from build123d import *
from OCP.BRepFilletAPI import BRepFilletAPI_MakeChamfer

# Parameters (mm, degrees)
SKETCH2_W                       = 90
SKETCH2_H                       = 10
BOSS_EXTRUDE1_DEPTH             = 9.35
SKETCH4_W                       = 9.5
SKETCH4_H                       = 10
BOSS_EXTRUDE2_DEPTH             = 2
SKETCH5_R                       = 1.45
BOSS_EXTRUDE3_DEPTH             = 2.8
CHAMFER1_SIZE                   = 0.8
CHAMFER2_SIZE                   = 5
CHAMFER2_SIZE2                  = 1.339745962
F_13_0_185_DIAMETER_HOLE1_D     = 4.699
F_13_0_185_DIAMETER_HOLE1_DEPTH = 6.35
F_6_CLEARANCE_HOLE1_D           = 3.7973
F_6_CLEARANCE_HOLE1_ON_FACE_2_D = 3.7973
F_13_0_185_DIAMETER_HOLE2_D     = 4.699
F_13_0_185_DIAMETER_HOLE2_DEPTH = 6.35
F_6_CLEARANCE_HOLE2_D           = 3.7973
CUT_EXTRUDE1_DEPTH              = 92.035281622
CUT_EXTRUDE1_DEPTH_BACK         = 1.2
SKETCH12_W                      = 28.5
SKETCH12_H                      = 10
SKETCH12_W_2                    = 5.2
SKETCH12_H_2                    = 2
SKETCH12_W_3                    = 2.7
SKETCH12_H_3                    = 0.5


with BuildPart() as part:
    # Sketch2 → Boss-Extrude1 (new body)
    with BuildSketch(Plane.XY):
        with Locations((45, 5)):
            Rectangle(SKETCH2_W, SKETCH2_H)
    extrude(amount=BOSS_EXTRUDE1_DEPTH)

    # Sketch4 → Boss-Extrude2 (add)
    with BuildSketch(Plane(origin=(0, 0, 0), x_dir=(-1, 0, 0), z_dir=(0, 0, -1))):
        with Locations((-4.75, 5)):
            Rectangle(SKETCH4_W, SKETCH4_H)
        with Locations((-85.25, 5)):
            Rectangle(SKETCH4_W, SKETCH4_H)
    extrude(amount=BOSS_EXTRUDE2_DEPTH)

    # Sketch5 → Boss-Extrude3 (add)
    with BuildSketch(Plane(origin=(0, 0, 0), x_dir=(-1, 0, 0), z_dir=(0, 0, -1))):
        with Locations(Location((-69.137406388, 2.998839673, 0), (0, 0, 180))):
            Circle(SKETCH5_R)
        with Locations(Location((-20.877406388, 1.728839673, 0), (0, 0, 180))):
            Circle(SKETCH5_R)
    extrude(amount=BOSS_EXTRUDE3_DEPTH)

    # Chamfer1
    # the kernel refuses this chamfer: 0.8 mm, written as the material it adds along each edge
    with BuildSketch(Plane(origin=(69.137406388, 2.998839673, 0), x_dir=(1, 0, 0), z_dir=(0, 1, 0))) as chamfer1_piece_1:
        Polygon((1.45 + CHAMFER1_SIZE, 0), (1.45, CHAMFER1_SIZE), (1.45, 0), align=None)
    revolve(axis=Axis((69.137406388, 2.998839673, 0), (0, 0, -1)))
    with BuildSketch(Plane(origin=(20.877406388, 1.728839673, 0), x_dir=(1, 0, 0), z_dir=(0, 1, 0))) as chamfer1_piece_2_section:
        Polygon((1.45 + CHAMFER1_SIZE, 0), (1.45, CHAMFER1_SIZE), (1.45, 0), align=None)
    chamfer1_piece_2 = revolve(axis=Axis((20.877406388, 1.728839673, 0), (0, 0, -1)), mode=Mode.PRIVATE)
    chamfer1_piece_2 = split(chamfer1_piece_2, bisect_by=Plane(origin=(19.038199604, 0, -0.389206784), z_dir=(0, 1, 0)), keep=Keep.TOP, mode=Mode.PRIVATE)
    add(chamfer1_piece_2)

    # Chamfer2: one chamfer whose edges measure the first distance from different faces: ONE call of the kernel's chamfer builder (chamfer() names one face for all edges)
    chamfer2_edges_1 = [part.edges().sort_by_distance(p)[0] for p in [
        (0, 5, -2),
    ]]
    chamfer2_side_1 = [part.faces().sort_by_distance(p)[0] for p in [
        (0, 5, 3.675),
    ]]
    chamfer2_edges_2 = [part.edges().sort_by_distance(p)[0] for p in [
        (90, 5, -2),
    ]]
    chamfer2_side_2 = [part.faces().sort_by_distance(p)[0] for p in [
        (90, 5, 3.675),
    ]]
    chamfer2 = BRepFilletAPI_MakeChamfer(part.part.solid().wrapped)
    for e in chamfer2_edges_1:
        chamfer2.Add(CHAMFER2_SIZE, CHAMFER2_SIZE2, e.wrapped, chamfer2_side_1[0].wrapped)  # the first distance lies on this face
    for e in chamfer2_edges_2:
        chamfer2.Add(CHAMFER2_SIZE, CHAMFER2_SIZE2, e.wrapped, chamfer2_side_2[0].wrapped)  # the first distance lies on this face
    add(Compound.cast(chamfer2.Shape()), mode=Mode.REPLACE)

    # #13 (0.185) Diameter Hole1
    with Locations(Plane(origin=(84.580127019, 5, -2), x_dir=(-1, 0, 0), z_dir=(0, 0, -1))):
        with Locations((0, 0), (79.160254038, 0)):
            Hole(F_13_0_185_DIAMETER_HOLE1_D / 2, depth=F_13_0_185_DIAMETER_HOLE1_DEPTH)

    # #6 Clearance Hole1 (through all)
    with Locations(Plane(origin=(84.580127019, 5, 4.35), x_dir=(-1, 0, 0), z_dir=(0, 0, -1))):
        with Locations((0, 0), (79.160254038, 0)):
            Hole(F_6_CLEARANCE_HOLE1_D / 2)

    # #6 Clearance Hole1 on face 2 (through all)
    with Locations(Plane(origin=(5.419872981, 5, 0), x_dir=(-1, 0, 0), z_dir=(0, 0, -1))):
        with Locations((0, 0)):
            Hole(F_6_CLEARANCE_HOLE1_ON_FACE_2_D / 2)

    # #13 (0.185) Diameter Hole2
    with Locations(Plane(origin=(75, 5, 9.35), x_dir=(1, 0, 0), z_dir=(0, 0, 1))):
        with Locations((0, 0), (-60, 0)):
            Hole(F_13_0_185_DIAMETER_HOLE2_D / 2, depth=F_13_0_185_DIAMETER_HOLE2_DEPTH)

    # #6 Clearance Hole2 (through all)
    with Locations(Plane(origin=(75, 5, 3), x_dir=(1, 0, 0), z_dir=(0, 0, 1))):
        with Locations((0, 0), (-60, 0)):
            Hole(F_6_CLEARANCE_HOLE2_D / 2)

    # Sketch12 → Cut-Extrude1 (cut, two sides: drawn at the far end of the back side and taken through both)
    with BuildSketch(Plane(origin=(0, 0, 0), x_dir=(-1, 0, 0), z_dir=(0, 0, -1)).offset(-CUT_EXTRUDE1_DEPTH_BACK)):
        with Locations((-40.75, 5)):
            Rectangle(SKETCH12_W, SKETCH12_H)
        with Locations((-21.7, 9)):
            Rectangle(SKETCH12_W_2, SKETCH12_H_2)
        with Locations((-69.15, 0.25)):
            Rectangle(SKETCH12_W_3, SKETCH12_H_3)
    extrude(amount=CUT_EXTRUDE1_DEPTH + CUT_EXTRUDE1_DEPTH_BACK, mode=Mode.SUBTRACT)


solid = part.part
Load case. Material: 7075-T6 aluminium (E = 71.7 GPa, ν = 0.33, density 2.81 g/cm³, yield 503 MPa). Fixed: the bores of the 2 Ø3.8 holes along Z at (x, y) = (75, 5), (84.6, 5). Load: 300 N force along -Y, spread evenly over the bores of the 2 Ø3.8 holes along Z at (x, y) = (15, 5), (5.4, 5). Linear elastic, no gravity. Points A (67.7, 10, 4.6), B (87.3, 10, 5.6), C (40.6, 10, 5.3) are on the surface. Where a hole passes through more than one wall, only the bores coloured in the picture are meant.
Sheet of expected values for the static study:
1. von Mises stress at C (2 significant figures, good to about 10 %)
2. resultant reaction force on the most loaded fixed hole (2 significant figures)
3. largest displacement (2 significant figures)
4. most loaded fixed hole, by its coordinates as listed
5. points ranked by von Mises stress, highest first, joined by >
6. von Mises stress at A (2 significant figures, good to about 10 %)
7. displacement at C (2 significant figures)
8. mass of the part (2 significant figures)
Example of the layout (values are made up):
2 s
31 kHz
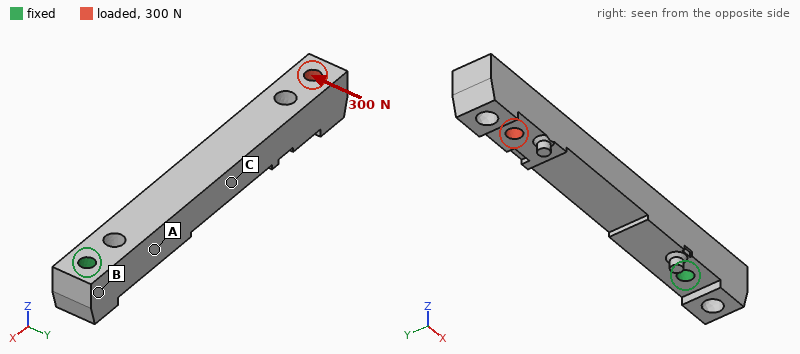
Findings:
70 MPa
1.2 kN
0.81 mm
(75, 5)
A > C > B
120 MPa
0.25 mm
22 g
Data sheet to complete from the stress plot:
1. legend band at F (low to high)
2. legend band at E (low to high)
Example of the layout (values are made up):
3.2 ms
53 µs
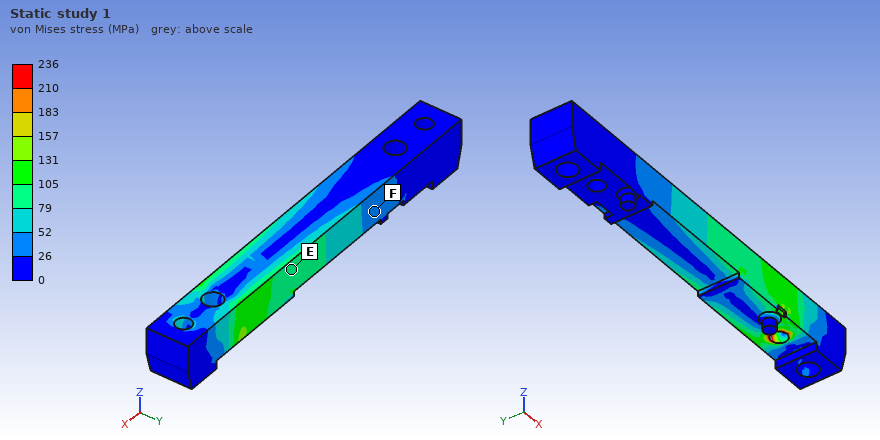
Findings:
26 to 52 MPa
79 to 105 MPa
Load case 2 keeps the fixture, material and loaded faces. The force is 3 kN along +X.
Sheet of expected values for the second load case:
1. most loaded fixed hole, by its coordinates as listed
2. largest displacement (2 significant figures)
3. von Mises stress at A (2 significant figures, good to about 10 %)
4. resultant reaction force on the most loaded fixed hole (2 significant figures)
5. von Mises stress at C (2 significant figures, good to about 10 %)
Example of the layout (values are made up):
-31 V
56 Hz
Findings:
(75, 5)
69 µm
34 MPa
1.7 kN
37 MPa
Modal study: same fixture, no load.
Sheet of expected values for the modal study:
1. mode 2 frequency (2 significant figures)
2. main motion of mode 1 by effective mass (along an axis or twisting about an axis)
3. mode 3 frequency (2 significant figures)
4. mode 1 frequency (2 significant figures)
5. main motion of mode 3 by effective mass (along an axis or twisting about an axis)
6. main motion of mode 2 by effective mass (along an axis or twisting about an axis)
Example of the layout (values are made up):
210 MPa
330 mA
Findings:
1300 Hz
along Z
6600 Hz
1200 Hz
along Z
along Y
